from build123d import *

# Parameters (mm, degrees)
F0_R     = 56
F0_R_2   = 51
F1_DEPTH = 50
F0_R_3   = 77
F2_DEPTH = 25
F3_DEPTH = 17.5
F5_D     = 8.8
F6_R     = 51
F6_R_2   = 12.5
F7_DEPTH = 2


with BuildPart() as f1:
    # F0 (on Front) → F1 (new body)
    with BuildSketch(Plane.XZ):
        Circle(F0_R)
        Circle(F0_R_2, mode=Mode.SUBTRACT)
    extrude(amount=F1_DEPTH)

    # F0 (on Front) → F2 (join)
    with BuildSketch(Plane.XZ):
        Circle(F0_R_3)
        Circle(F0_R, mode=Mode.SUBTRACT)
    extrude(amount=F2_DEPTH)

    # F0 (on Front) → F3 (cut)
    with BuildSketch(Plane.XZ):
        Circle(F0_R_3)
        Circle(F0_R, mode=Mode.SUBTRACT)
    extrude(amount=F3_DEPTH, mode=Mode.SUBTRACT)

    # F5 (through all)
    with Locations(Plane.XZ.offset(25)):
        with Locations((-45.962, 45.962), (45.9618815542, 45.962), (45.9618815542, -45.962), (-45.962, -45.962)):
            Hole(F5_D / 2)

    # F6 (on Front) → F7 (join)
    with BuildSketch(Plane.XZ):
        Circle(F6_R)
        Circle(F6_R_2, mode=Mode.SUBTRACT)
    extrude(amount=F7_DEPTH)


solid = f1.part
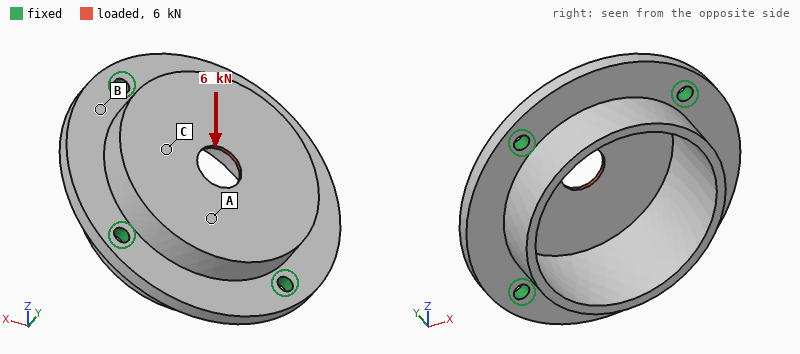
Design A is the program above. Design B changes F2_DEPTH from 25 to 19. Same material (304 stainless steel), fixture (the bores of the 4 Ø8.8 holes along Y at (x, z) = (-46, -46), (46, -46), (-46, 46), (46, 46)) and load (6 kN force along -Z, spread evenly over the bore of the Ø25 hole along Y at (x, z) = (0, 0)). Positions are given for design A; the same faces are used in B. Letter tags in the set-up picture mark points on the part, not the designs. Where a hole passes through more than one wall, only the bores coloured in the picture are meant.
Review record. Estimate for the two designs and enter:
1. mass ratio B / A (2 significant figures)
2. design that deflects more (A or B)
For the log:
0.69
B
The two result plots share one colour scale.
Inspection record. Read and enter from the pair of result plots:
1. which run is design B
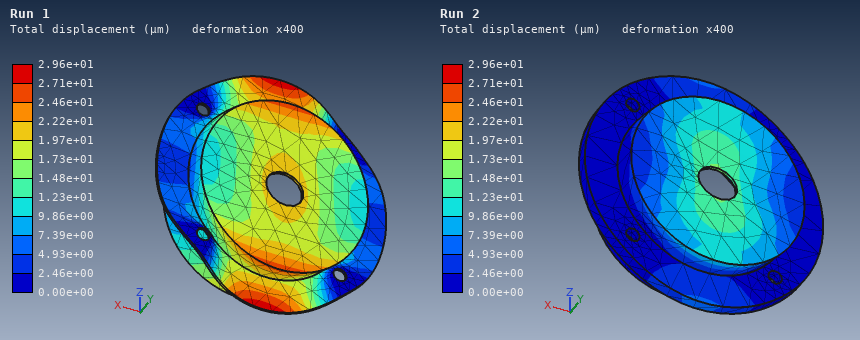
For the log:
Run 1
